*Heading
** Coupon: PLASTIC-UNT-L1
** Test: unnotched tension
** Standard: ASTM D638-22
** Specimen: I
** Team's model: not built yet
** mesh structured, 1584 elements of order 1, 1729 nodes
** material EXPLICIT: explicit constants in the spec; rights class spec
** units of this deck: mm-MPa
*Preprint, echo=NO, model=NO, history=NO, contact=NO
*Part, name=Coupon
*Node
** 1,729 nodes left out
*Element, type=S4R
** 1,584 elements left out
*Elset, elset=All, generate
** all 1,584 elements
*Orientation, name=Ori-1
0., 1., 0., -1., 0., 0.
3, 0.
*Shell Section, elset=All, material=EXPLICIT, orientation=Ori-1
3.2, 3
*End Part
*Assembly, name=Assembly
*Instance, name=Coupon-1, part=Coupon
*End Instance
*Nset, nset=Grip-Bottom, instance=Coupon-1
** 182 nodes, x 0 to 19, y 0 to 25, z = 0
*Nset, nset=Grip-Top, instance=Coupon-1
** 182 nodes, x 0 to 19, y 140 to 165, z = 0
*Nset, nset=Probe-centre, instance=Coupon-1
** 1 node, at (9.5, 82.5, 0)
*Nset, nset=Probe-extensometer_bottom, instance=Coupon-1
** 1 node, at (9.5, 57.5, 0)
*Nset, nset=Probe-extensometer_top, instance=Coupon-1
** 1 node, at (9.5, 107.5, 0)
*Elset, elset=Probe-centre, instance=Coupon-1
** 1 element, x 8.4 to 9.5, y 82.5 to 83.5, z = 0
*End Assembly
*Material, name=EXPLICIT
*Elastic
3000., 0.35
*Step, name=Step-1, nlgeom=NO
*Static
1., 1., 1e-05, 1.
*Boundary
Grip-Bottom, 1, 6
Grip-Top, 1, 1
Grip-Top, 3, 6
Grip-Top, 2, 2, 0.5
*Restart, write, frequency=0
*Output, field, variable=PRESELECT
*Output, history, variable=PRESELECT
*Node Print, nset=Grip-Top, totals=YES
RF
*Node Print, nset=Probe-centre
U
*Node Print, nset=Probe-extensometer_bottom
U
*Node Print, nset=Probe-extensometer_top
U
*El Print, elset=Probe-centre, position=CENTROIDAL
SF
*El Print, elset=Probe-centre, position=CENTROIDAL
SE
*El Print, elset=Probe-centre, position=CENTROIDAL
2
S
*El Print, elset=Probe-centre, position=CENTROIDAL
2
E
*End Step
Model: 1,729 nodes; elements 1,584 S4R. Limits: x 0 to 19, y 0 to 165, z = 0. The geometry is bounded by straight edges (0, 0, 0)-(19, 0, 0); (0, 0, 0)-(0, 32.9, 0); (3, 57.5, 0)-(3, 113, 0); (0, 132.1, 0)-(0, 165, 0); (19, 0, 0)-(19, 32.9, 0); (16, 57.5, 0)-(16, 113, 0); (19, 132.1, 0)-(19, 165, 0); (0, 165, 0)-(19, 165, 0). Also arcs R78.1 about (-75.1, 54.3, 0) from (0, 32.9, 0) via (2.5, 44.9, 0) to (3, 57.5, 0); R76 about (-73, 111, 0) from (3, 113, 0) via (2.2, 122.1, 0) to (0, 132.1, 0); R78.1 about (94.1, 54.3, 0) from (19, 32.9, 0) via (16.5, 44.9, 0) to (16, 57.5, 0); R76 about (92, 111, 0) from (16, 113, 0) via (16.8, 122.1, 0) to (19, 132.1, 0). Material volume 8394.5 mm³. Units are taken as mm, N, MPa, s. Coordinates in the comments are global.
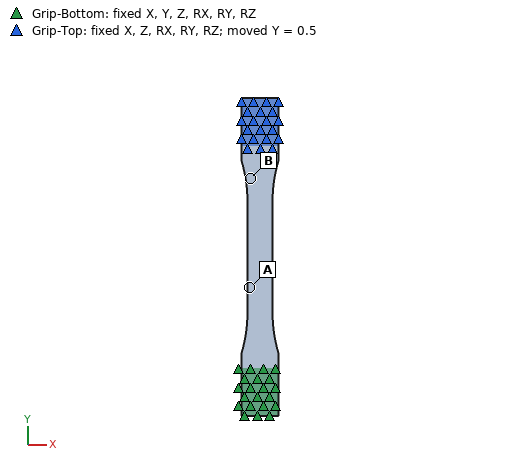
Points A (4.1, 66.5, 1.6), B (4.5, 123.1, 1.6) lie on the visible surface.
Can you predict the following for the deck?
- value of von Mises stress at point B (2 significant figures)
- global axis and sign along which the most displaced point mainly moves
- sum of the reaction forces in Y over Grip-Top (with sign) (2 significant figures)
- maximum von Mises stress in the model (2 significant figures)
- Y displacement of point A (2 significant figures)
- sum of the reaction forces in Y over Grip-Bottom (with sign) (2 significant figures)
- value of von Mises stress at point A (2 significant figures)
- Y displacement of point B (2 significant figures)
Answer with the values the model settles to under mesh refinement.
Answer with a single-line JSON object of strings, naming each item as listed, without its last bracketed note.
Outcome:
{"value of von Mises stress at point B": "12 MPa", "global axis and sign along which the most displaced point mainly moves": "+Y", "sum of the reaction forces in Y over Grip-Top (with sign)": "600 N", "maximum von Mises stress in the model": "15 MPa", "Y displacement of point A": "0.17 mm", "sum of the reaction forces in Y over Grip-Bottom (with sign)": "-600 N", "value of von Mises stress at point A": "14 MPa", "Y displacement of point B": "0.44 mm"}
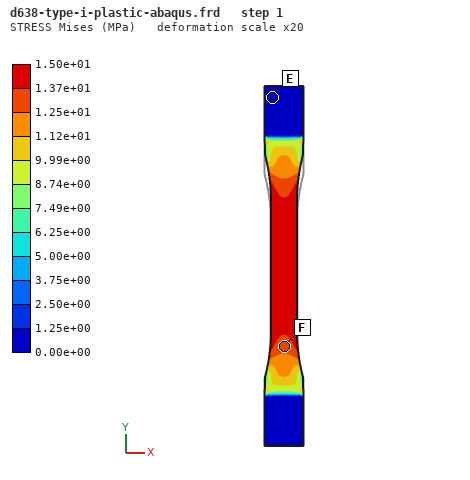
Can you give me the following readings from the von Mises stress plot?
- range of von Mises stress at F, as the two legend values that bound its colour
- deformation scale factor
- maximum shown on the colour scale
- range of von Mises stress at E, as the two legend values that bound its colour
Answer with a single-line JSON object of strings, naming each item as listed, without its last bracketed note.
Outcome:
{"range of von Mises stress at F, as the two legend values that bound its colour": "1.25e+01 to 1.37e+01 MPa", "deformation scale factor": "20", "maximum shown on the colour scale": "1.50e+01 MPa", "range of von Mises stress at E, as the two legend values that bound its colour": "0.00e+00 to 1.25e+00 MPa"}
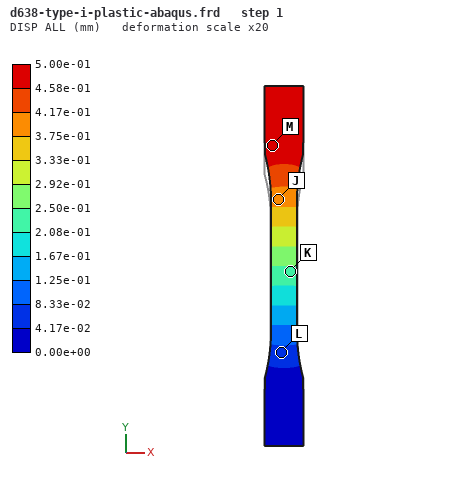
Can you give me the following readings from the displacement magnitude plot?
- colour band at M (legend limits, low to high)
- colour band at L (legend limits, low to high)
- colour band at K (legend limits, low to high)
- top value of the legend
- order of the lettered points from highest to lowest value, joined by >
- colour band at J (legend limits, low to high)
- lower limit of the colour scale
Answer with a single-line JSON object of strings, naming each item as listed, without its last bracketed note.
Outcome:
{"colour band at M": "4.58e-01 to 5.00e-01 mm", "colour band at L": "4.17e-02 to 8.33e-02 mm", "colour band at K": "2.08e-01 to 2.50e-01 mm", "top value of the legend": "5.00e-01 mm", "order of the lettered points from highest to lowest value, joined by >": "M > J > K > L", "colour band at J": "3.75e-01 to 4.17e-01 mm", "lower limit of the colour scale": "0.00e+00 mm"}
